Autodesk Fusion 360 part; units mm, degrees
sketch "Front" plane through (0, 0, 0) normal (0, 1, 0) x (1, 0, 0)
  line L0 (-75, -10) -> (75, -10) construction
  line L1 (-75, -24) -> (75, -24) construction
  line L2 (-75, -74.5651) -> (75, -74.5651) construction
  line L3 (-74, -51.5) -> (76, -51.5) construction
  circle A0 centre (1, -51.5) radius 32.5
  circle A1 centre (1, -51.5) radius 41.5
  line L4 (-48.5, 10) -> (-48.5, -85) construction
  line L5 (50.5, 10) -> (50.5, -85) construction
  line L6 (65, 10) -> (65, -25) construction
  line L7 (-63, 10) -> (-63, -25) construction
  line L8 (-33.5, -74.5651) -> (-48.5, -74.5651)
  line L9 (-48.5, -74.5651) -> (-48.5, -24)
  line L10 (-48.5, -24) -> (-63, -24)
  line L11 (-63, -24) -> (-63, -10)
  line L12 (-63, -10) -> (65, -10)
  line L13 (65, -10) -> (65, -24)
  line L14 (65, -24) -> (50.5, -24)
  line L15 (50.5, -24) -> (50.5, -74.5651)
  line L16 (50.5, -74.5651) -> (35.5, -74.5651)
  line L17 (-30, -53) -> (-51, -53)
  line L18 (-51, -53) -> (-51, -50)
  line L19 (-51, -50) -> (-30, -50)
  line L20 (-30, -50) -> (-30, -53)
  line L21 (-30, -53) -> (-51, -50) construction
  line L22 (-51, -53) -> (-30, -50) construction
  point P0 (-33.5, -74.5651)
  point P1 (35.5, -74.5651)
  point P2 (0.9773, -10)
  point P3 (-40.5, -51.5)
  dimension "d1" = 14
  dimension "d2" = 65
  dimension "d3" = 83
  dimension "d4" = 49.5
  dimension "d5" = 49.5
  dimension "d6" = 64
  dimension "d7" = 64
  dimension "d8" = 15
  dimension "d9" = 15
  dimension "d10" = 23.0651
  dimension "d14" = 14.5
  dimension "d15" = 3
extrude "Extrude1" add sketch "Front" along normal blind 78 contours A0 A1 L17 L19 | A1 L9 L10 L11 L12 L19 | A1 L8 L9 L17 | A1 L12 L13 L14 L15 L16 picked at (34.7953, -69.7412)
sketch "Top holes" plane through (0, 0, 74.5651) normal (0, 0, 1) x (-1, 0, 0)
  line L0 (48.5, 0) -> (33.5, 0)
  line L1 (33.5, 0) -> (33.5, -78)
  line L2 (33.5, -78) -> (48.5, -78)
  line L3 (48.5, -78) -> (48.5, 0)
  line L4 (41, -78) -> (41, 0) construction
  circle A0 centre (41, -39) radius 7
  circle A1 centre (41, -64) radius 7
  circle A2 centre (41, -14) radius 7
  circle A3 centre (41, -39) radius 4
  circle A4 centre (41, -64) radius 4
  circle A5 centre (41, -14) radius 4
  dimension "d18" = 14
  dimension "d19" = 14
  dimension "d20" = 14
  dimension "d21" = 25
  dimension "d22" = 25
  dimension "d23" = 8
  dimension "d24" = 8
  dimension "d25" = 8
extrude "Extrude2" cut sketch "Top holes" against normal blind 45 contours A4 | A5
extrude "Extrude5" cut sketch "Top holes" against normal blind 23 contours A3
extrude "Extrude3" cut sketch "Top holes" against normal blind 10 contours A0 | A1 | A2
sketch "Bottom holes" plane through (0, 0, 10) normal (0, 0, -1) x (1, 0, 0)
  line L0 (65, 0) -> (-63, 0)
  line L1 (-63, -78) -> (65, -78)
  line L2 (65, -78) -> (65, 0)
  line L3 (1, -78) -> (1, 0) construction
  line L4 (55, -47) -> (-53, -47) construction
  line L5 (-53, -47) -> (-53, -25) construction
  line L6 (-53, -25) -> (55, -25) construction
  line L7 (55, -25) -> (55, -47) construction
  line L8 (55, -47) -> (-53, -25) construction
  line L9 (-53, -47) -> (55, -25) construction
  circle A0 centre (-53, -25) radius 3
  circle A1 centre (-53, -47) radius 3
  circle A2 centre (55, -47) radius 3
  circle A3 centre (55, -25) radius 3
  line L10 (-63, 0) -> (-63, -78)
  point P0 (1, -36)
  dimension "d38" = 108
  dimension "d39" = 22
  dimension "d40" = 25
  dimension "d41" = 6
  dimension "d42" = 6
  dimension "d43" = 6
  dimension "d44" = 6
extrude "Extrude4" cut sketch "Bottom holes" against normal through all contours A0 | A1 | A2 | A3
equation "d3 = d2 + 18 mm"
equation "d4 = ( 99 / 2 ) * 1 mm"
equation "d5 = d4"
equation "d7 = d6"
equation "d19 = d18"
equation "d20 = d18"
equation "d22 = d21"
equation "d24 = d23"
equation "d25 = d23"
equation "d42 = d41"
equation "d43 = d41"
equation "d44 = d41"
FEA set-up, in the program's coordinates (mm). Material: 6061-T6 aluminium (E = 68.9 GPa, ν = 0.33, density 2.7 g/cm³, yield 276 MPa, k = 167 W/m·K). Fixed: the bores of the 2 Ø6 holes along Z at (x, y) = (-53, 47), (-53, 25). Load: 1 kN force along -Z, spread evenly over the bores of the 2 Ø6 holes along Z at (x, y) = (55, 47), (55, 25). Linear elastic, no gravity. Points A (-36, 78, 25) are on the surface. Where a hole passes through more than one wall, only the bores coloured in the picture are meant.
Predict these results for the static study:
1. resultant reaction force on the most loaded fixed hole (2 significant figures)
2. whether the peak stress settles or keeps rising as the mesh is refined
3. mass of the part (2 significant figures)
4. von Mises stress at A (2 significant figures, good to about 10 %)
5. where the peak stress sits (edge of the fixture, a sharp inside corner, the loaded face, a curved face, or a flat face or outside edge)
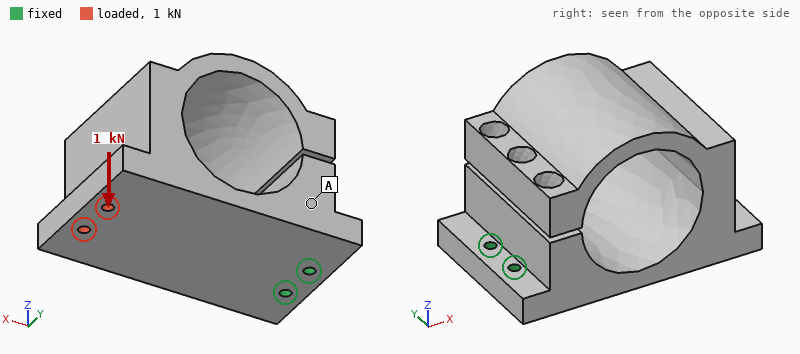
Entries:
520 N
keeps rising
880 g
8.5 MPa
edge of the fixture
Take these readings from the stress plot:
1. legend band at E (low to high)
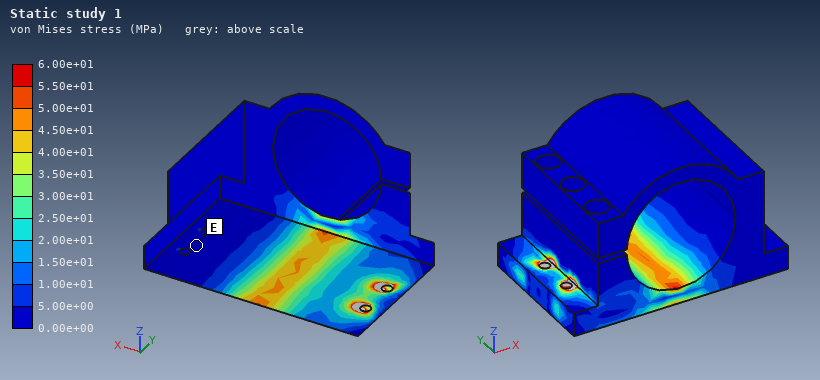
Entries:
0.00e+00 to 5.00e+00 MPa
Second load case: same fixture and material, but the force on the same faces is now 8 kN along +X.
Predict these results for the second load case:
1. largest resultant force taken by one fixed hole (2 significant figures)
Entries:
4.0 kN
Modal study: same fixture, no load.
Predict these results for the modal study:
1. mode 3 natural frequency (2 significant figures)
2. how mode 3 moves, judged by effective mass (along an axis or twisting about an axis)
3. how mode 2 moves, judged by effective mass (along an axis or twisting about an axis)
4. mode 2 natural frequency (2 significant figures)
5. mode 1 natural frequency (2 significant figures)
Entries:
650 Hz
along Y
along Z
620 Hz
350 Hz
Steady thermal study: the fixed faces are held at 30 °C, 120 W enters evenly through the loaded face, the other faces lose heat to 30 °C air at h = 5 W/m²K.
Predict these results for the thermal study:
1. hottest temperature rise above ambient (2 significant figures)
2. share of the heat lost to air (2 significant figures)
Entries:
74 K
11 %
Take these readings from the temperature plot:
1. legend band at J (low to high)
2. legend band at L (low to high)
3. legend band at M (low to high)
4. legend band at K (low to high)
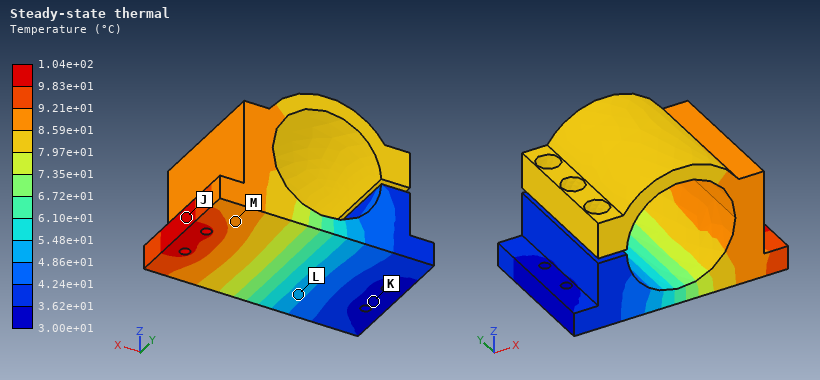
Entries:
9.83e+01 to 1.04e+02 °C
4.86e+01 to 5.48e+01 °C
8.59e+01 to 9.21e+01 °C
3.00e+01 to 3.62e+01 °C
